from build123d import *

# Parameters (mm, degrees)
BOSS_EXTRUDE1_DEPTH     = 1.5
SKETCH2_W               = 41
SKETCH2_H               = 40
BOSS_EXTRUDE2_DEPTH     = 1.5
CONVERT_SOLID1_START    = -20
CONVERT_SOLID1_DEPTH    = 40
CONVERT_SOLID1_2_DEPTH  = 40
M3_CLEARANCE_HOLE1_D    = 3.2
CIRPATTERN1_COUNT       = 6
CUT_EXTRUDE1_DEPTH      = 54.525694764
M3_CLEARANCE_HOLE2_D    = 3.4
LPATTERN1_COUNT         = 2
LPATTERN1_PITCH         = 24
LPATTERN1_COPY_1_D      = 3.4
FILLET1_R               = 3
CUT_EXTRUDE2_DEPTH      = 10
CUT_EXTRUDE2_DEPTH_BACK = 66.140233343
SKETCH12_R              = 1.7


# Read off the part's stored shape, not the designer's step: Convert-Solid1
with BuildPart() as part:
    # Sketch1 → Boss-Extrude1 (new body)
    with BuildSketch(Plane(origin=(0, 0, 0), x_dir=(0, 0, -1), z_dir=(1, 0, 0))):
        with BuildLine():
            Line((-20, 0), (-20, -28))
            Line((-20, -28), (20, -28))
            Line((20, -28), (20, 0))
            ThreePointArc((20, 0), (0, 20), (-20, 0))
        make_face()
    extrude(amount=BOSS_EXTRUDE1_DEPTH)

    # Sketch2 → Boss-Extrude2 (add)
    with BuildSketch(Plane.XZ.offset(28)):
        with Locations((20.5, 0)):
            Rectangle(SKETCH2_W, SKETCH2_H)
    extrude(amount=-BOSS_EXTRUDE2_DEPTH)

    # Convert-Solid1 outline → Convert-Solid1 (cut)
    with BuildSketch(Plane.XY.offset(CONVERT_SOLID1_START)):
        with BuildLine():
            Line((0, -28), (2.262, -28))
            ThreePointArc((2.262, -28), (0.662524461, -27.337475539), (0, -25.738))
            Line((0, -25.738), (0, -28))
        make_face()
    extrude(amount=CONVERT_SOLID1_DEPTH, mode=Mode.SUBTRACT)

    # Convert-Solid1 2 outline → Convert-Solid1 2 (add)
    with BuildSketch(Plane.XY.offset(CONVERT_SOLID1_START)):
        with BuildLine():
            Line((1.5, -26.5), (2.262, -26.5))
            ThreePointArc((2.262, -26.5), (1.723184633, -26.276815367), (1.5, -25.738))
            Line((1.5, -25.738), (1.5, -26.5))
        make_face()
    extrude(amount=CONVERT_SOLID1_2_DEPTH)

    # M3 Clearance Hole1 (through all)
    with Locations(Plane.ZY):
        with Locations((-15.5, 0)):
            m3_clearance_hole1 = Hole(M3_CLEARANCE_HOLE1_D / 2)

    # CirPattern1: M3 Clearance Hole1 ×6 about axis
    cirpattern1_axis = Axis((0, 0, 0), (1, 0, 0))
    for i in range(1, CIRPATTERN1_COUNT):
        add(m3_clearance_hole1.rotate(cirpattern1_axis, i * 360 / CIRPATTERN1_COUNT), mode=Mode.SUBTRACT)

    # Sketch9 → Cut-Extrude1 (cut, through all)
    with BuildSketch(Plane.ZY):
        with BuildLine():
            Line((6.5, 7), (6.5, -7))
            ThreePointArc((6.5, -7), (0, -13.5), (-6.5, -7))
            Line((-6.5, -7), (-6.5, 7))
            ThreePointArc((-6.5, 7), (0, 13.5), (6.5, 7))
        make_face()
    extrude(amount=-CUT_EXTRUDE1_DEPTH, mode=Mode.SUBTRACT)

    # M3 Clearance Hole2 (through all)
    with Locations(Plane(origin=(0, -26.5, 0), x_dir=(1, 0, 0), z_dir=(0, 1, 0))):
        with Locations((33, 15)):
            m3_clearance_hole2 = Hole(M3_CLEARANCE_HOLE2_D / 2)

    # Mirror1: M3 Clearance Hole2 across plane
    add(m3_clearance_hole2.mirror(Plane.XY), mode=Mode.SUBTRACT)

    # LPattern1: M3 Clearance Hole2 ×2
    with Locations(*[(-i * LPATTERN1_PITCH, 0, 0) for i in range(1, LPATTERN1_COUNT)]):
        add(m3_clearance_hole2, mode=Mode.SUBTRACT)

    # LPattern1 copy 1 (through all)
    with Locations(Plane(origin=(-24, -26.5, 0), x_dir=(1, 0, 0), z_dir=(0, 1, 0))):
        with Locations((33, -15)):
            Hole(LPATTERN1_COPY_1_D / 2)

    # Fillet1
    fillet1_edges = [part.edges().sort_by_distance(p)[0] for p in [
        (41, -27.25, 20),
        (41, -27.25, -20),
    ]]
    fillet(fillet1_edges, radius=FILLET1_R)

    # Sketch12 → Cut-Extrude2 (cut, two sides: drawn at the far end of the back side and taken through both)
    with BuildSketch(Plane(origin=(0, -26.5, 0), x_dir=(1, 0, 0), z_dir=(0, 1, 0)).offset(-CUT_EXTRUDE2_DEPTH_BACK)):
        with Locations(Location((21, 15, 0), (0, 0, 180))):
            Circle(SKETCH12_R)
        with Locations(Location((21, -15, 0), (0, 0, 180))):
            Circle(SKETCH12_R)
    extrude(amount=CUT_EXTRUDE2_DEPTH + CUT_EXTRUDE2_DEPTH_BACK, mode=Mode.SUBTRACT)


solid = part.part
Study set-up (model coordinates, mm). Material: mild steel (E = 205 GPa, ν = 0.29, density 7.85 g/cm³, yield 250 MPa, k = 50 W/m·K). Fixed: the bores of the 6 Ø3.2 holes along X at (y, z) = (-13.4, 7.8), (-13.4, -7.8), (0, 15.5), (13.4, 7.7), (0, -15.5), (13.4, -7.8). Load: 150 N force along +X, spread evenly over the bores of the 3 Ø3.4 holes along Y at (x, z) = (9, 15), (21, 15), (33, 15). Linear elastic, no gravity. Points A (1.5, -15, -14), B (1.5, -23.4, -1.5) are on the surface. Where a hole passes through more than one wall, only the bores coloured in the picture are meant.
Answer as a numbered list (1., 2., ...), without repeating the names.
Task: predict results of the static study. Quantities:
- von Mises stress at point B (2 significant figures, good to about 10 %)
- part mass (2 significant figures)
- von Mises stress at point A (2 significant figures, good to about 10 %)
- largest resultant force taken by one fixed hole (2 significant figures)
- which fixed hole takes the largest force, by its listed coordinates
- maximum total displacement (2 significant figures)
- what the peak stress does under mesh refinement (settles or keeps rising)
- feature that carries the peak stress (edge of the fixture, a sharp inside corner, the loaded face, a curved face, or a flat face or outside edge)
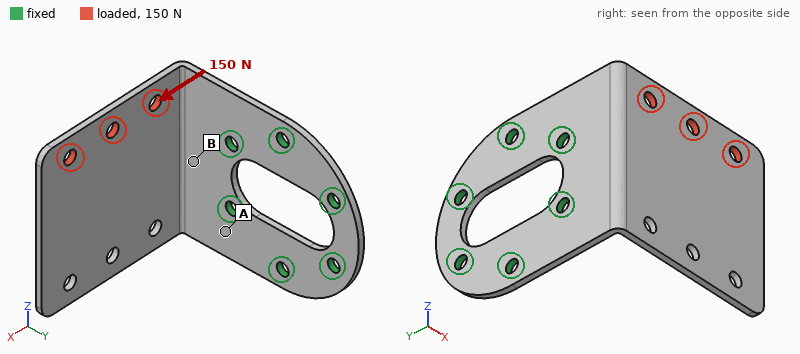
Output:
1. 76 MPa
2. 34 g
3. 30 MPa
4. 200 N
5. (-13.4, 7.8)
6. 0.33 mm
7. keeps rising
8. edge of the fixture
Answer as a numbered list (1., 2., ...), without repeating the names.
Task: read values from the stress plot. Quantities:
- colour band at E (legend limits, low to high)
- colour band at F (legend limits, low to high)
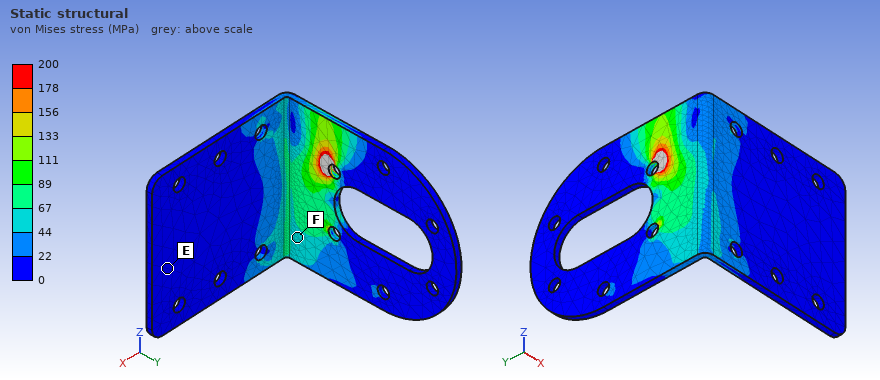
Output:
1. 0 to 22 MPa
2. 44 to 67 MPa
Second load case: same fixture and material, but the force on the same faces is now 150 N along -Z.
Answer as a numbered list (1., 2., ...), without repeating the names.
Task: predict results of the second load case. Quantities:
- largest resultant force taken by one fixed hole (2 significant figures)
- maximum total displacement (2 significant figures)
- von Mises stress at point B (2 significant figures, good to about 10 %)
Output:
1. 180 N
2. 0.21 mm
3. 100 MPa
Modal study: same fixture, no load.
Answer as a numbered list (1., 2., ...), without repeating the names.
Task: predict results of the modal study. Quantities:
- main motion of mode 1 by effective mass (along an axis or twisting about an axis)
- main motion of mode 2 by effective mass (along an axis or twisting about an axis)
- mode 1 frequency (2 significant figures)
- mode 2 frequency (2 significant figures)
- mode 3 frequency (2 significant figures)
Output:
1. along Y
2. along Z
3. 510 Hz
4. 1100 Hz
5. 1900 Hz
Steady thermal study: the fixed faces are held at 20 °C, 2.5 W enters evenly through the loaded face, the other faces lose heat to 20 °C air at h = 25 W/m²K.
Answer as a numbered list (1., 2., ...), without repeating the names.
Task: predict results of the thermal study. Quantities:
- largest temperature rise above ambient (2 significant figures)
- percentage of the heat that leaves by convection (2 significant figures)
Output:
1. 24 K
2. 49 %
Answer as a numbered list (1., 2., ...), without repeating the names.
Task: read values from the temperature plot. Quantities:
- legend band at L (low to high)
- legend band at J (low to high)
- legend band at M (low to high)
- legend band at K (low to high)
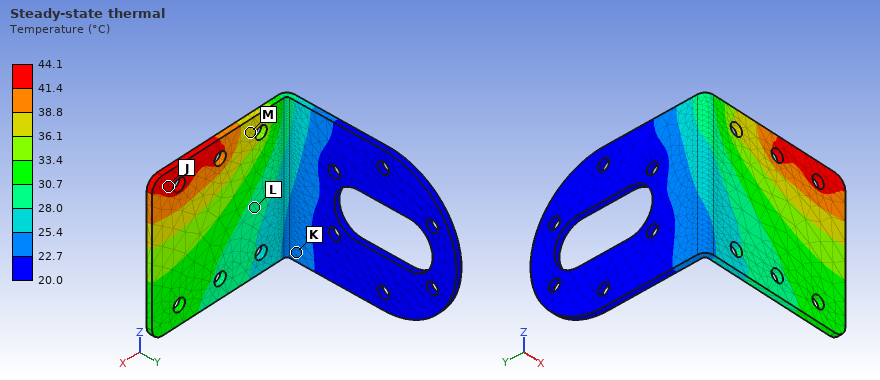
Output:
1. 28.0 to 30.7 °C
2. 41.4 to 44.1 °C
3. 36.1 to 38.8 °C
4. 22.7 to 25.4 °C
